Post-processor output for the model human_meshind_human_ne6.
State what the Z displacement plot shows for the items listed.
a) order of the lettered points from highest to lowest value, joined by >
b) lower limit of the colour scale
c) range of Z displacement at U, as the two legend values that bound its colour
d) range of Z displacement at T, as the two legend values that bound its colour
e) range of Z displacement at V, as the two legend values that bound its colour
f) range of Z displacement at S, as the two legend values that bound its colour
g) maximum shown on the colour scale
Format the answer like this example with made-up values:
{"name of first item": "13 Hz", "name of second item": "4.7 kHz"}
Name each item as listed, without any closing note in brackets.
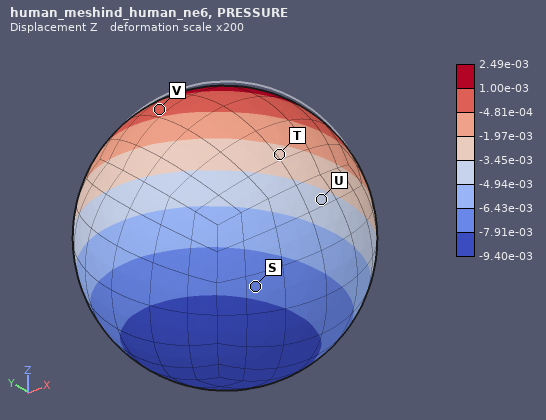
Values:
{"order of the lettered points from highest to lowest value, joined by >": "V > T > U > S", "lower limit of the colour scale": "-9.40e-03", "range of Z displacement at U, as the two legend values that bound its colour": "-4.94e-03 to -3.45e-03", "range of Z displacement at T, as the two legend values that bound its colour": "-3.45e-03 to -1.97e-03", "range of Z displacement at V, as the two legend values that bound its colour": "-4.81e-04 to 1.00e-03", "range of Z displacement at S, as the two legend values that bound its colour": "-7.91e-03 to -6.43e-03", "maximum shown on the colour scale": "2.49e-03"}
